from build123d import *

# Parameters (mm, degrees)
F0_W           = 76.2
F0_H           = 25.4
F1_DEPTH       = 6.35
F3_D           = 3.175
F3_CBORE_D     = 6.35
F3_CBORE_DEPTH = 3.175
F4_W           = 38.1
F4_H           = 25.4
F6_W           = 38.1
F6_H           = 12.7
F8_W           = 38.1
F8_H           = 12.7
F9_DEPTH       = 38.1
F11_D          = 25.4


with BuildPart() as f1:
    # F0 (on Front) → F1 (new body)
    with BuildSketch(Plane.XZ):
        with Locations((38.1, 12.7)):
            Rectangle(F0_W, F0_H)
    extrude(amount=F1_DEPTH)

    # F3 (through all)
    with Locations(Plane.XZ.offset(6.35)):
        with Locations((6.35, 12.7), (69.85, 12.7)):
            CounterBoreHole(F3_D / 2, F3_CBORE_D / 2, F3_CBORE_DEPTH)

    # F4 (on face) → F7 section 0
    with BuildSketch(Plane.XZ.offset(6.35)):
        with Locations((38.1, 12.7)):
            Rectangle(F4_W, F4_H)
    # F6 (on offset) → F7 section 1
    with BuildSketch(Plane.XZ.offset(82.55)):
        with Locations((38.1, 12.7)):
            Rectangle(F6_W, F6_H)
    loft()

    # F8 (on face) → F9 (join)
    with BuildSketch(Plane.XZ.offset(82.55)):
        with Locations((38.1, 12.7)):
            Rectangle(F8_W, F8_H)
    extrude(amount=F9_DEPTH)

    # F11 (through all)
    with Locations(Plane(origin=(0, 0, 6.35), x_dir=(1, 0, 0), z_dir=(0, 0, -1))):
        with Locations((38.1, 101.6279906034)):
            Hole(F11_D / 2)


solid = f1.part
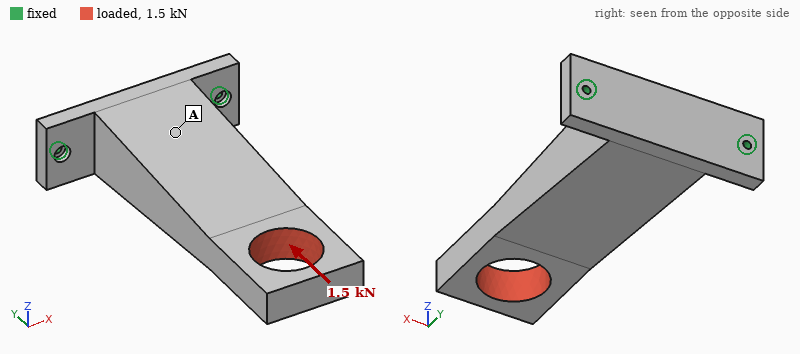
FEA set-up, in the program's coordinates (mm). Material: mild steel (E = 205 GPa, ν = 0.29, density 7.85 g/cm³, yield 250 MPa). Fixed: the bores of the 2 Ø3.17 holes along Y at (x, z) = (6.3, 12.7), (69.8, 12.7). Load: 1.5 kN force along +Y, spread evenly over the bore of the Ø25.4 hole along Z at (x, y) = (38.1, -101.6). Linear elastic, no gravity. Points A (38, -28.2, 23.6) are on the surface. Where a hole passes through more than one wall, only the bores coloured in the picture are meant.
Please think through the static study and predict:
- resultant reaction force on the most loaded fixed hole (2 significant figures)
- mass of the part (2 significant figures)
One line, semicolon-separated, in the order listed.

1.1 kN; 620 g
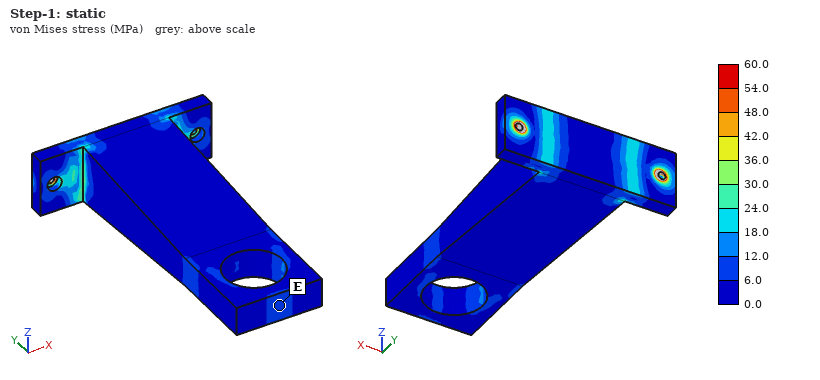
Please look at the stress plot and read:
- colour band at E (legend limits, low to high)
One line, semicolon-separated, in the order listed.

6.0 to 12.0 MPa
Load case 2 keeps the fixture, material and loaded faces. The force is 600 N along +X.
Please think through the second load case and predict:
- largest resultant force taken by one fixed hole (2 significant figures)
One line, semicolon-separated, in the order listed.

1.1 kN
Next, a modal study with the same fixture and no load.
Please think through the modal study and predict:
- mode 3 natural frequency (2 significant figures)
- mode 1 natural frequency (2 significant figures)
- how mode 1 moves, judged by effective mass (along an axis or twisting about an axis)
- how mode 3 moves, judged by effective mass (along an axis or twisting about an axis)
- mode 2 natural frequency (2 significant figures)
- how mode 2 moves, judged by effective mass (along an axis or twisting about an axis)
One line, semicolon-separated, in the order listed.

3000 Hz; 330 Hz; along Z; along Y; 1400 Hz; along X
